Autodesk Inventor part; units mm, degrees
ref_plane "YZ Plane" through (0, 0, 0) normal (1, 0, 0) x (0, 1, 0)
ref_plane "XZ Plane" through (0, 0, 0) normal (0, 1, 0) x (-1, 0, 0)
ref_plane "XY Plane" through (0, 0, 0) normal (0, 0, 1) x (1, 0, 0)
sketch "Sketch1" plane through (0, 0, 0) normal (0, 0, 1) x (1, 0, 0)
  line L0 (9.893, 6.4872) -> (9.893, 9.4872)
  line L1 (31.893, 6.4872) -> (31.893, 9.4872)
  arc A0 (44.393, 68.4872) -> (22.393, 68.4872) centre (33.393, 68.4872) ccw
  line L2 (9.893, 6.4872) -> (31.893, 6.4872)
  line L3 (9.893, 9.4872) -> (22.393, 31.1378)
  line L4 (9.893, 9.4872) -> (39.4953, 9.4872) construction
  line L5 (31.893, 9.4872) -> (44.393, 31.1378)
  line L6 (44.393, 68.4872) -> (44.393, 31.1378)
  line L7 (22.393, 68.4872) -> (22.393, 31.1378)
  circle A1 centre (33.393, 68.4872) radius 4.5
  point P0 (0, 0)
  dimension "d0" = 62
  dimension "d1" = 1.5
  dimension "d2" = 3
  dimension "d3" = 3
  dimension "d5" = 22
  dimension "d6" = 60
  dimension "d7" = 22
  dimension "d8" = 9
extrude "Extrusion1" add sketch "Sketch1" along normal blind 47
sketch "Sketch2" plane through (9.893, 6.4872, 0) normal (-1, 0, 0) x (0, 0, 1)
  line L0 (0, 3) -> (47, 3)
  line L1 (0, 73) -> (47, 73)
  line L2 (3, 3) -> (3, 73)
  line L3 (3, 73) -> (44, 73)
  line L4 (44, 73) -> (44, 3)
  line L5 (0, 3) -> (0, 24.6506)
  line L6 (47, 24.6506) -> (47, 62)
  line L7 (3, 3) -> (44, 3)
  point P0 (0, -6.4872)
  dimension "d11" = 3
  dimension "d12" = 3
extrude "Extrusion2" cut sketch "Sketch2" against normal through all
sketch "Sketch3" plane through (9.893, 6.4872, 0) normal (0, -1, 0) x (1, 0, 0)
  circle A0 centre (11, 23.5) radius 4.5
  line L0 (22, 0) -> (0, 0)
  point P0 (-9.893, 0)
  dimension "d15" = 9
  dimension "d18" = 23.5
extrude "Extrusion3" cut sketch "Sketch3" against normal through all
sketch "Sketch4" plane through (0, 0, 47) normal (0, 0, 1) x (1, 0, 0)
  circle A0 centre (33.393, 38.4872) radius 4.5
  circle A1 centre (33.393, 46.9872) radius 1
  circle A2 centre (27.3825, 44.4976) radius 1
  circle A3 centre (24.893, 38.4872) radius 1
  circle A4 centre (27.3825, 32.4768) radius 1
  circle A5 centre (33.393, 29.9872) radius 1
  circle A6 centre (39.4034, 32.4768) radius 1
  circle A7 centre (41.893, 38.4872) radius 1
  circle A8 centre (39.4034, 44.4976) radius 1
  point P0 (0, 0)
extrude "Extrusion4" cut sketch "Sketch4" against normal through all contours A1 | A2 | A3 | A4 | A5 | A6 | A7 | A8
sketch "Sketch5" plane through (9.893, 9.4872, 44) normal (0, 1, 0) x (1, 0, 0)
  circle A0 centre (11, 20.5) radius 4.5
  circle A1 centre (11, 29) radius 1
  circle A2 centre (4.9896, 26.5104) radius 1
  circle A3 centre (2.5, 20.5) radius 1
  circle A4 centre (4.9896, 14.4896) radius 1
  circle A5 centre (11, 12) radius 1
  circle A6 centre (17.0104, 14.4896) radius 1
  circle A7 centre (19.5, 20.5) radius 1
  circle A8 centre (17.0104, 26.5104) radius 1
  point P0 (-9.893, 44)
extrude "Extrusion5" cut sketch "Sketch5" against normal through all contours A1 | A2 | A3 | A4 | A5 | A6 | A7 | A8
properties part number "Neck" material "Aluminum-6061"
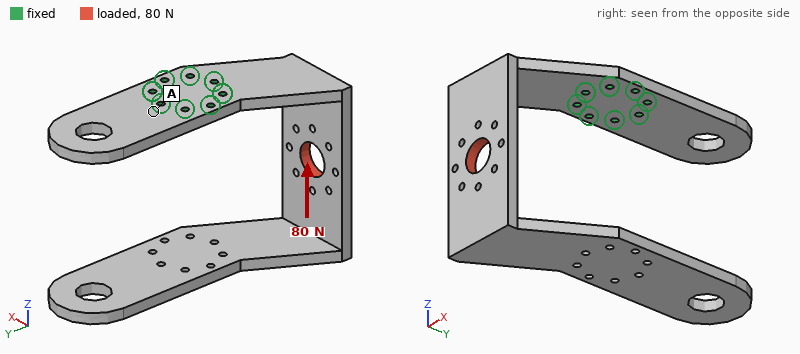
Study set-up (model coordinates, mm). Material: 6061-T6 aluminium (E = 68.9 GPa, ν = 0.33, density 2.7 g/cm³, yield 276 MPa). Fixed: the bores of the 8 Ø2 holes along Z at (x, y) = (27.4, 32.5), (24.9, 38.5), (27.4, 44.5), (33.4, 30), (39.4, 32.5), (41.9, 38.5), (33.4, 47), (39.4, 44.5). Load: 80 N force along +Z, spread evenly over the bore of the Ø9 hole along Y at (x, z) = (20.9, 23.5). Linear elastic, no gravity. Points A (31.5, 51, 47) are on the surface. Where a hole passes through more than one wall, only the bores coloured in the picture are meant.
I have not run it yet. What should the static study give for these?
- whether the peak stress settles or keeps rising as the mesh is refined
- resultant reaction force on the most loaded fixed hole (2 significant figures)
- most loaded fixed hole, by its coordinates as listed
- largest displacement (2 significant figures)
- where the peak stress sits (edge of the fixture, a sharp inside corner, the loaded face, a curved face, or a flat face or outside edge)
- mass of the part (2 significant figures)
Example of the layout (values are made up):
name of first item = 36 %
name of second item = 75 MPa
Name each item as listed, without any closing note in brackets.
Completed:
whether the peak stress settles or keeps rising as the mesh is refined = keeps rising
resultant reaction force on the most loaded fixed hole = 120 N
most loaded fixed hole, by its coordinates as listed = (33.4, 30)
largest displacement = 0.58 mm
where the peak stress sits = edge of the fixture
mass of the part = 30 g
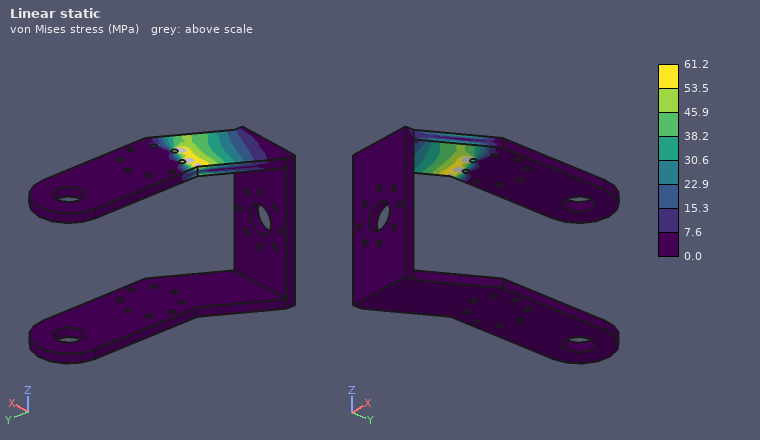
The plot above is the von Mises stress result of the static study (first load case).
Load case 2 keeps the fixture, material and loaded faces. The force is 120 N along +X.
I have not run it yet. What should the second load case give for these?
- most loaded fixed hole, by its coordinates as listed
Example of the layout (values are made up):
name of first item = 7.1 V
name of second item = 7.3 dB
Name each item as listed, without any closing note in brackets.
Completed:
most loaded fixed hole, by its coordinates as listed = (27.4, 32.5)
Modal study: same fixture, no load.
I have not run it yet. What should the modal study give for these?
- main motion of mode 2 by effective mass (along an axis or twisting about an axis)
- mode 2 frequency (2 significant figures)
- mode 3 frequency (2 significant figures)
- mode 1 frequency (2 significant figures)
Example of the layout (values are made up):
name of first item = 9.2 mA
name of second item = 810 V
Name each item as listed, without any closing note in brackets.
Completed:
main motion of mode 2 by effective mass = along X
mode 2 frequency = 290 Hz
mode 3 frequency = 500 Hz
mode 1 frequency = 190 Hz
